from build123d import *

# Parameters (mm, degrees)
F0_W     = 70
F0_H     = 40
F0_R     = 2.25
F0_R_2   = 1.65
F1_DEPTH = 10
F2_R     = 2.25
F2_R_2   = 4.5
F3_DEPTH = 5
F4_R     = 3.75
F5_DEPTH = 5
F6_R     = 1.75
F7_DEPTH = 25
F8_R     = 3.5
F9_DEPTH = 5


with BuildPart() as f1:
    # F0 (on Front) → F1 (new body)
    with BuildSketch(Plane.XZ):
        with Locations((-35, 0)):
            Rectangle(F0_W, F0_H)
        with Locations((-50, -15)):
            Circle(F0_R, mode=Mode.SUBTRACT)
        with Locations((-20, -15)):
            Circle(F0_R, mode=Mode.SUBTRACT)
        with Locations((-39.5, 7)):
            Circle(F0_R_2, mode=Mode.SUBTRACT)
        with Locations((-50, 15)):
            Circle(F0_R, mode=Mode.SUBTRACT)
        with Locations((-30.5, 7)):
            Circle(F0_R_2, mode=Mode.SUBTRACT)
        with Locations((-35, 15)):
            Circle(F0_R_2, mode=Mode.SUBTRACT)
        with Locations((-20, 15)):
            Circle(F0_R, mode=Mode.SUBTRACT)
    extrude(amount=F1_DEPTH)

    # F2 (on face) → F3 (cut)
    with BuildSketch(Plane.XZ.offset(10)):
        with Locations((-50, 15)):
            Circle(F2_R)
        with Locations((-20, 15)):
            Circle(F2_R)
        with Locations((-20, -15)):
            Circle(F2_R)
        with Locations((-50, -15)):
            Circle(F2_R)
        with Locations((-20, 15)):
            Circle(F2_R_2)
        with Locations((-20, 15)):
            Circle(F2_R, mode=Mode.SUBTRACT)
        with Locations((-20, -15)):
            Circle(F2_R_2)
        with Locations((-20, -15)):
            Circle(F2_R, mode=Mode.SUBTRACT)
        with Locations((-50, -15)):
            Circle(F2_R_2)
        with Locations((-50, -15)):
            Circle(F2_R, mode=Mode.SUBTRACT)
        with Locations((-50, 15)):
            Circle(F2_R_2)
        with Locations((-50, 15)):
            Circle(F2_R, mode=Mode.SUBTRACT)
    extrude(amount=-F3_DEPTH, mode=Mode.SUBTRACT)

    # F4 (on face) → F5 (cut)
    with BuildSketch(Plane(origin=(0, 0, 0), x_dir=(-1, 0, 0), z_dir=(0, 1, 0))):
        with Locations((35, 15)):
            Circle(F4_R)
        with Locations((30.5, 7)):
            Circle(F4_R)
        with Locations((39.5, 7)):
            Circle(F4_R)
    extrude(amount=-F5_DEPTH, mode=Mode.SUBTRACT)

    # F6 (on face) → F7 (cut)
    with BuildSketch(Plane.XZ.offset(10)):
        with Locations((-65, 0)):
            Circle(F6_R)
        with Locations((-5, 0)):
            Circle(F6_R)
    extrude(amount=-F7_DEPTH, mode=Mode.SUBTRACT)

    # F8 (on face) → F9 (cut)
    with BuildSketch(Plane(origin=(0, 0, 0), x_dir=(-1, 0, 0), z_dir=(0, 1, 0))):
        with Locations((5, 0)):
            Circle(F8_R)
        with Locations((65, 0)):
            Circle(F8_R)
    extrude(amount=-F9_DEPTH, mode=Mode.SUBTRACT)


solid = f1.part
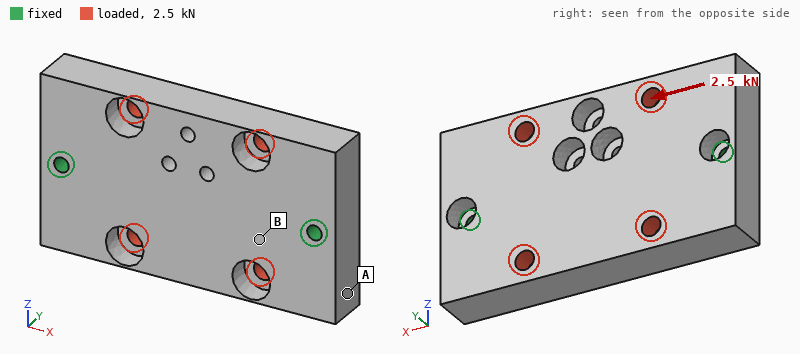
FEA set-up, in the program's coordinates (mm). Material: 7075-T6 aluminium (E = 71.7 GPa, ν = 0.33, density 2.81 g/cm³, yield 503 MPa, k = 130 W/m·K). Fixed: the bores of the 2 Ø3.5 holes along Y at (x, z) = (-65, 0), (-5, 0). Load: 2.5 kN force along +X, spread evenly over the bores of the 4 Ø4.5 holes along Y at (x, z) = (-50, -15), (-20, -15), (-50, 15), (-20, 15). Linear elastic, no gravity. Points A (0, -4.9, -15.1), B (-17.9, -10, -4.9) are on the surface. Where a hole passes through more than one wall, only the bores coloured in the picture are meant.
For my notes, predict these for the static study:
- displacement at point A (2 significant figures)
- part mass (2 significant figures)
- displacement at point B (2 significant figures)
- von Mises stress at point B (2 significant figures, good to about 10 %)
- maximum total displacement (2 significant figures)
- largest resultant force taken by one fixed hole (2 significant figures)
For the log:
3.2 µm
71 g
2.4 µm
8.3 MPa
4.5 µm
1.3 kN
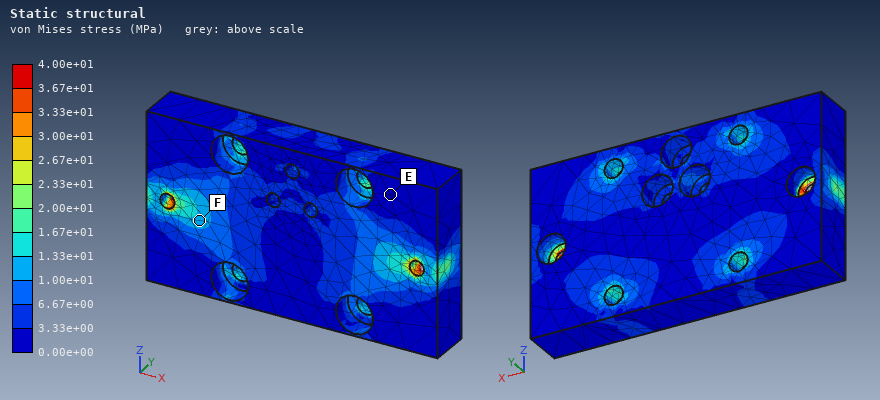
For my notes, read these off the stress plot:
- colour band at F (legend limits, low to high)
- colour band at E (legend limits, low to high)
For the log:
1.00e+01 to 1.33e+01 MPa
0.00e+00 to 3.33e+00 MPa
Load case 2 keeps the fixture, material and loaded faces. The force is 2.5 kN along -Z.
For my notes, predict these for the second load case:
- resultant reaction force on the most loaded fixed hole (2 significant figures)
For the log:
1.3 kN
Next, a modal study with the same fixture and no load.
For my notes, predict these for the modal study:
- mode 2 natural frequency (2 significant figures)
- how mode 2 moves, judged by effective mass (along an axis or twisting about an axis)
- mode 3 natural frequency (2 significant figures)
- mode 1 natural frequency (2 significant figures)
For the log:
6900 Hz
along Y
11 kHz
4800 Hz
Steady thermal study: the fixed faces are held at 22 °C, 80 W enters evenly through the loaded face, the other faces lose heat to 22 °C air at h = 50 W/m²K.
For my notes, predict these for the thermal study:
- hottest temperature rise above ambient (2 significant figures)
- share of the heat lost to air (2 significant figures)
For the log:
32 K
11 %
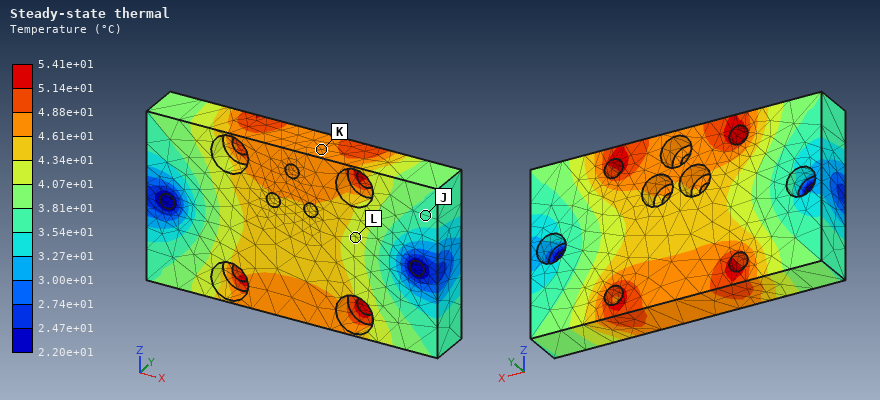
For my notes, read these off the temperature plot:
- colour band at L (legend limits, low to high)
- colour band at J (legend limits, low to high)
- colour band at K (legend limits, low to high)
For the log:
4.07e+01 to 4.34e+01 °C
3.54e+01 to 3.81e+01 °C
4.61e+01 to 4.88e+01 °C
